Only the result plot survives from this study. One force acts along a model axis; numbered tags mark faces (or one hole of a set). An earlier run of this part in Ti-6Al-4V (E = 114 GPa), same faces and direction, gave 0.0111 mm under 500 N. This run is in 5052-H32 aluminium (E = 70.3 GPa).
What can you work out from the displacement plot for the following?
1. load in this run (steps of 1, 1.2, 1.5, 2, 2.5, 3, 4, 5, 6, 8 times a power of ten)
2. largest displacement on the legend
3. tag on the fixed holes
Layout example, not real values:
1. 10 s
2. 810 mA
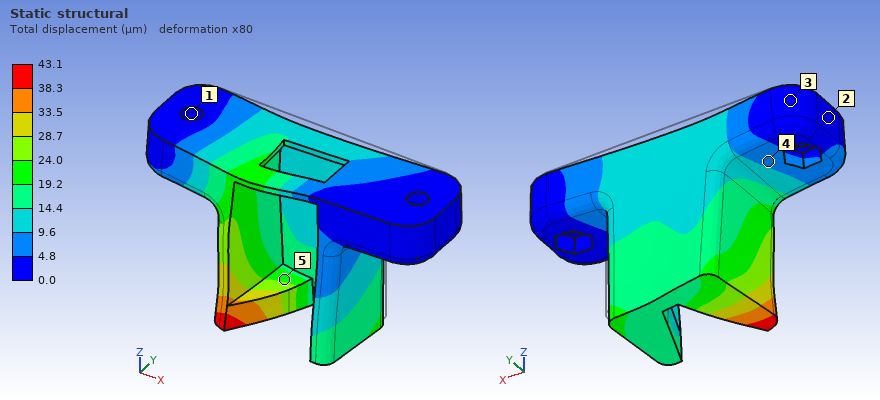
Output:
1. 1.2 kN
2. 43.1 µm
3. 1
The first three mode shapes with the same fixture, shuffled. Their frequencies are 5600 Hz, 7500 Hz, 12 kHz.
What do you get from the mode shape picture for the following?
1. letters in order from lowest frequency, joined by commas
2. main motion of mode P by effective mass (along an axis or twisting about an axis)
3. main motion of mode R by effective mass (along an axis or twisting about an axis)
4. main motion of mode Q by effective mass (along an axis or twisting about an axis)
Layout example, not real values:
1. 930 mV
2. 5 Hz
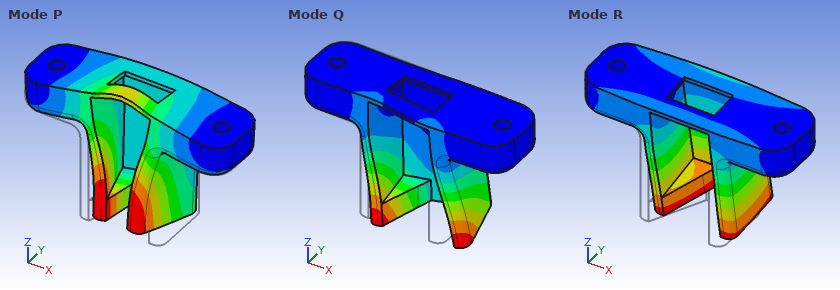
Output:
1. R, Q, P
2. along Z
3. along Y
4. along X
